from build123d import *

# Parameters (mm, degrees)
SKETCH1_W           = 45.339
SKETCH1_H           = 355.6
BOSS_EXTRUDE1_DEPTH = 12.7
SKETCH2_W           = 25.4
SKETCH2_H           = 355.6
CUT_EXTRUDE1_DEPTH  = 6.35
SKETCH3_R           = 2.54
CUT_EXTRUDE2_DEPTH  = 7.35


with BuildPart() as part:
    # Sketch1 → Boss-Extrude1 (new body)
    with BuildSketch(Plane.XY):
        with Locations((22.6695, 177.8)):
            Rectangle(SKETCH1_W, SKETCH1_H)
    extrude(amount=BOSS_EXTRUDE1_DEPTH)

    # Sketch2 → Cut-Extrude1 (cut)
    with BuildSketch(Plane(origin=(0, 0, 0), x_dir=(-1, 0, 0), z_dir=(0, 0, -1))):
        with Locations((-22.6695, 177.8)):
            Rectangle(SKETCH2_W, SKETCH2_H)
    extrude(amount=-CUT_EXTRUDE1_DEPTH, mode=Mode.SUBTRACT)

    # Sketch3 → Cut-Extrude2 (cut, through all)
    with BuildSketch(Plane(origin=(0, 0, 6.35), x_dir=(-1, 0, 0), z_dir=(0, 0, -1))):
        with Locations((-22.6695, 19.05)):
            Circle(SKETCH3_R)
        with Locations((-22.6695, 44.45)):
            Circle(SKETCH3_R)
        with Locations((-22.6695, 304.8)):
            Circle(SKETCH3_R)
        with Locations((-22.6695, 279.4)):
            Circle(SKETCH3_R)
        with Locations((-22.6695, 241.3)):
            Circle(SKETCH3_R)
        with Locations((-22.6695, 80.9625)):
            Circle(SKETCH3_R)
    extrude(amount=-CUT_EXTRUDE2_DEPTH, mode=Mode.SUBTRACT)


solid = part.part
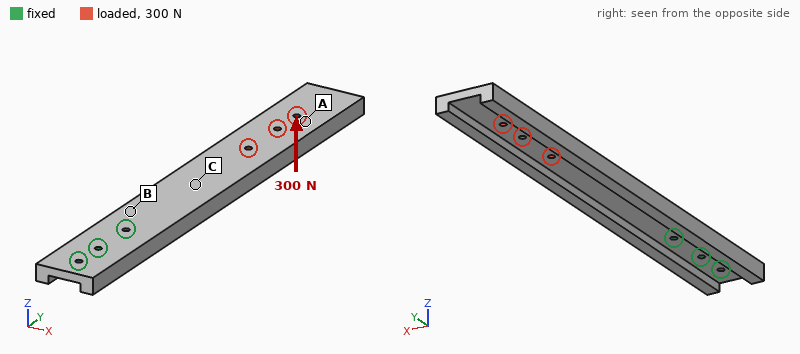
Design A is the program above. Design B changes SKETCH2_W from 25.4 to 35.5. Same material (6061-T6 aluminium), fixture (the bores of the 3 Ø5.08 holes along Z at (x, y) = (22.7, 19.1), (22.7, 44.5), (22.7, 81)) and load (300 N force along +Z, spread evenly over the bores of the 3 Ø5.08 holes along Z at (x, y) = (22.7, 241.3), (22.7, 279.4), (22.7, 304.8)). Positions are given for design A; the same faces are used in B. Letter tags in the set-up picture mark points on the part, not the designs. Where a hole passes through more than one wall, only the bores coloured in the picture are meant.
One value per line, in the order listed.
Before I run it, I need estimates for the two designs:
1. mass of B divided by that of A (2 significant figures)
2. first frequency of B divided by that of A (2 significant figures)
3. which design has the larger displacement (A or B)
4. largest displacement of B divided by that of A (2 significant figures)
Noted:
0.84
0.89
B
1.5
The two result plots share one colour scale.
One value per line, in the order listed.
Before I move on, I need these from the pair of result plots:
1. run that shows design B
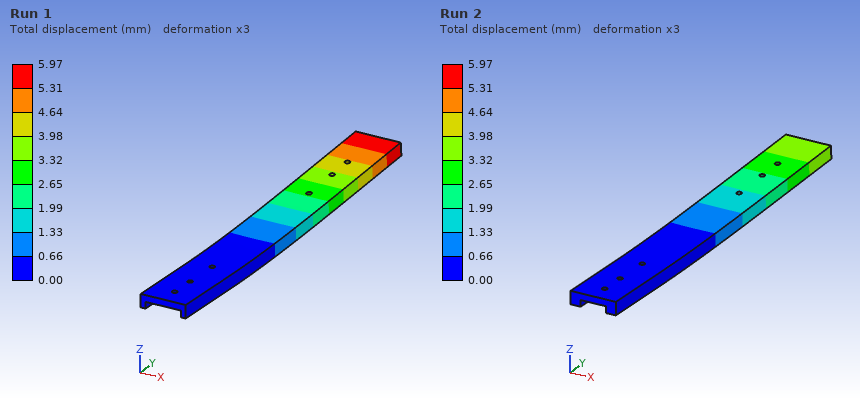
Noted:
Run 1
